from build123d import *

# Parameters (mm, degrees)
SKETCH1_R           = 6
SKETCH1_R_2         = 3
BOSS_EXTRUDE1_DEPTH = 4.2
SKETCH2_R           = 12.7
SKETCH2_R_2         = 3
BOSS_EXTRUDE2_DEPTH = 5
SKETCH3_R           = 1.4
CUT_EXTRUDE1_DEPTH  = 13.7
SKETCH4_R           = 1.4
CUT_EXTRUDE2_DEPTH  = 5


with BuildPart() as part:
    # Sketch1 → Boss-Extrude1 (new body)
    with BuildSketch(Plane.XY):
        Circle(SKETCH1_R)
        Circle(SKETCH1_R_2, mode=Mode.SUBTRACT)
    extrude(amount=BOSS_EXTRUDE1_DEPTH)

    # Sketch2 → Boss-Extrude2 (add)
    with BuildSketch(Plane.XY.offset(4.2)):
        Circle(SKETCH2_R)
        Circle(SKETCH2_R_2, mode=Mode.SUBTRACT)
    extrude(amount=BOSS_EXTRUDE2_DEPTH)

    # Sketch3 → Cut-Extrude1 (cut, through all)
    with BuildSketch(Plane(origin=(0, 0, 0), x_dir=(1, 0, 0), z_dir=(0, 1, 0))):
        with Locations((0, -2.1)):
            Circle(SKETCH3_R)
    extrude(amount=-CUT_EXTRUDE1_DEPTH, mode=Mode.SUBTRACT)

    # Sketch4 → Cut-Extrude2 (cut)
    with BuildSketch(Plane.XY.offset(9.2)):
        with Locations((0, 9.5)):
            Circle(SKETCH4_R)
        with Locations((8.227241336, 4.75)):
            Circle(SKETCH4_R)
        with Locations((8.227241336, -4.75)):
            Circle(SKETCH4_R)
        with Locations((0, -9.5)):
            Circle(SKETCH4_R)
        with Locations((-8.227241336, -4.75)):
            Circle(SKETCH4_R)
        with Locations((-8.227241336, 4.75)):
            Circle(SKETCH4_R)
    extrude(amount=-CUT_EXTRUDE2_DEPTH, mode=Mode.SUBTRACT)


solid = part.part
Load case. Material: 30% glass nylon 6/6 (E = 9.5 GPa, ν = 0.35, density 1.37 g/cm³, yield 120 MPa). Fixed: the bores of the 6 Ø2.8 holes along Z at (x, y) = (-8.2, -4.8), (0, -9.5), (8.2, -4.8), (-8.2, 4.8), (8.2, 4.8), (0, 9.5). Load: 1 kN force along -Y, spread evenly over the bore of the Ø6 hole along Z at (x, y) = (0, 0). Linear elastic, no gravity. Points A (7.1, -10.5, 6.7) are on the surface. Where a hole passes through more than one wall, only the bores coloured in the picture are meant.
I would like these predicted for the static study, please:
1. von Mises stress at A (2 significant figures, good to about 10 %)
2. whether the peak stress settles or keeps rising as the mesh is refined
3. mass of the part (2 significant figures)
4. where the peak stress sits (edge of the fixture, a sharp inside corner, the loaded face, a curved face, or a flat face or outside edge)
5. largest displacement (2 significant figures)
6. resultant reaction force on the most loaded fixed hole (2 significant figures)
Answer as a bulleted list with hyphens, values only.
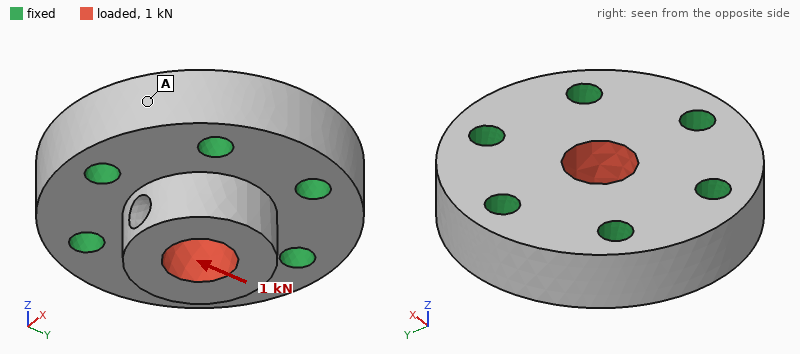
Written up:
- 2.2 MPa
- keeps rising
- 3.5 g
- a sharp inside corner
- 16 µm
- 280 N
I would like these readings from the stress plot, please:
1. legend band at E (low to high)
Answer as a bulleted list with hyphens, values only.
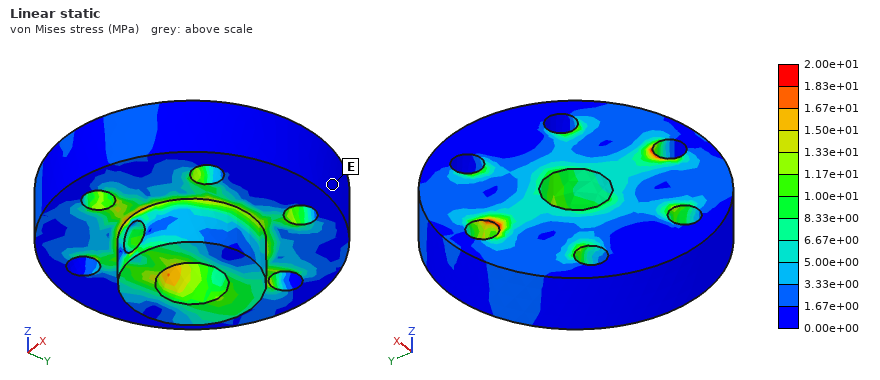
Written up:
- 0.00e+00 to 1.67e+00 MPa
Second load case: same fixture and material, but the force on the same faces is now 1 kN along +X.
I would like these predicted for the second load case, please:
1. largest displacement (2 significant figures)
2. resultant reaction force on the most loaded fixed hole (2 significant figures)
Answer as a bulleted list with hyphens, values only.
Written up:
- 17 µm
- 250 N
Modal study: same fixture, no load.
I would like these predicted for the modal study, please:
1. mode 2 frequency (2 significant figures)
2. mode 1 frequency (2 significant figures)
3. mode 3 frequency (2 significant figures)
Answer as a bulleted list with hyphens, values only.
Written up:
- 48 kHz
- 47 kHz
- 49 kHz
